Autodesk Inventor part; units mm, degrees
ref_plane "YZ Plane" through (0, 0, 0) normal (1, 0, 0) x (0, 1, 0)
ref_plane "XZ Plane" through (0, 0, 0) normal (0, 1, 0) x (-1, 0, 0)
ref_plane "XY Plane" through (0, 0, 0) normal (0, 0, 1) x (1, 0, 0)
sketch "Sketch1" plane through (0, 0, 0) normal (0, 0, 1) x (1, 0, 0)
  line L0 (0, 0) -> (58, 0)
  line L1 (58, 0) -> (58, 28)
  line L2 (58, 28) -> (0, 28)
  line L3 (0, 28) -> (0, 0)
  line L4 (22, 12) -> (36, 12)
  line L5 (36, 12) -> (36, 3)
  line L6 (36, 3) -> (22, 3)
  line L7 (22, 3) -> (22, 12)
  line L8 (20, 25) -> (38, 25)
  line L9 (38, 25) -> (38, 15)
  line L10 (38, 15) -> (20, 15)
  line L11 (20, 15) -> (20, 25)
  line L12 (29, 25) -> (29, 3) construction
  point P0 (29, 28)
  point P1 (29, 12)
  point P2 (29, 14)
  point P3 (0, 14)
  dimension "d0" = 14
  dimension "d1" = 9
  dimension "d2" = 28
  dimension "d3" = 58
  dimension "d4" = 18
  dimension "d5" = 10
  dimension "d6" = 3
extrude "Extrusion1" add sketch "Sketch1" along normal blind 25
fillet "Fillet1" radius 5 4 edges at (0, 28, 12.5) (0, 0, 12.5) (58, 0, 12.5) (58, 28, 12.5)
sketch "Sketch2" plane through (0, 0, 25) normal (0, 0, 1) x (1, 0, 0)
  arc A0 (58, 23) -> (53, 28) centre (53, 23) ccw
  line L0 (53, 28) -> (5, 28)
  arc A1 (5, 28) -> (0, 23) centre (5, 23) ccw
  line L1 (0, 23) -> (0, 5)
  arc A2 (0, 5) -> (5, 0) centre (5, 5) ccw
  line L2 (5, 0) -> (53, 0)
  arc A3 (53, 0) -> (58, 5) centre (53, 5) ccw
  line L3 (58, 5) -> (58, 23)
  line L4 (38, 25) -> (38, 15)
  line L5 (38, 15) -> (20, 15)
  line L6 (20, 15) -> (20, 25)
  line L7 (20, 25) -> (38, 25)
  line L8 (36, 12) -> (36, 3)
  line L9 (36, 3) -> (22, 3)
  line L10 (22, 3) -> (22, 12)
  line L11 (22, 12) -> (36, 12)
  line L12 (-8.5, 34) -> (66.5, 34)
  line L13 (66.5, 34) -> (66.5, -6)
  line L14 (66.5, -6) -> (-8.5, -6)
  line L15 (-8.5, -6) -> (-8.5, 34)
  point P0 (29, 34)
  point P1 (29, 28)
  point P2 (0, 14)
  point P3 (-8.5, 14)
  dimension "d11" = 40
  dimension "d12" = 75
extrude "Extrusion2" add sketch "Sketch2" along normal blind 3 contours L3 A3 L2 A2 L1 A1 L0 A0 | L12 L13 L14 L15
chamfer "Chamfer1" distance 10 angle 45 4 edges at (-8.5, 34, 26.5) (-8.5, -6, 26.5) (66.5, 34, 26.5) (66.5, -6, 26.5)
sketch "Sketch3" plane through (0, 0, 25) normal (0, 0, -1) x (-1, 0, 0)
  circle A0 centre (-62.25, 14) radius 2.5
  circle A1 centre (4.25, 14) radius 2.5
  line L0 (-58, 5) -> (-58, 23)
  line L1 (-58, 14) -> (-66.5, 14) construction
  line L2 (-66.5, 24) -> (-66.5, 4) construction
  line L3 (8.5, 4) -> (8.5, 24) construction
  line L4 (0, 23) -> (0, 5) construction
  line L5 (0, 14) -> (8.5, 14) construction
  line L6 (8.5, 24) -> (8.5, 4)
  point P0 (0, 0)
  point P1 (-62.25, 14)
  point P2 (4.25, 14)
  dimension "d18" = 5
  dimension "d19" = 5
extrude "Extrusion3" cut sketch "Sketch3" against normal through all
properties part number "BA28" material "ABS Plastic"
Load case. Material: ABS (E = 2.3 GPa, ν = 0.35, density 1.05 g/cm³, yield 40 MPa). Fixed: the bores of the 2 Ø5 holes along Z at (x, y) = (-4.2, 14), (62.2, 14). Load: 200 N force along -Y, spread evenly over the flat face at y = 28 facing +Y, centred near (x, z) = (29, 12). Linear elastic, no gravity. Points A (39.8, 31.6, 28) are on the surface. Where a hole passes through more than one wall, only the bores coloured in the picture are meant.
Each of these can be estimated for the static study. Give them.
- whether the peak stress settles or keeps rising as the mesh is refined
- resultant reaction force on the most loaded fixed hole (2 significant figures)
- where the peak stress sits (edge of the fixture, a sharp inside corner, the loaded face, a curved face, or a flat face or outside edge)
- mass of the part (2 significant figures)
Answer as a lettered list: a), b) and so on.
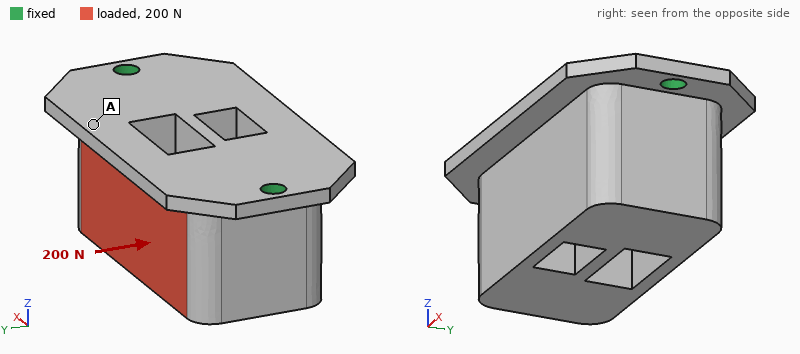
a) keeps rising
b) 100 N
c) edge of the fixture
d) 42 g
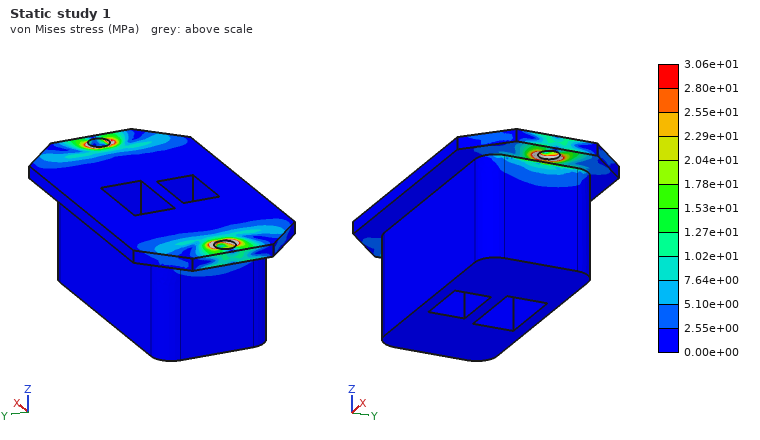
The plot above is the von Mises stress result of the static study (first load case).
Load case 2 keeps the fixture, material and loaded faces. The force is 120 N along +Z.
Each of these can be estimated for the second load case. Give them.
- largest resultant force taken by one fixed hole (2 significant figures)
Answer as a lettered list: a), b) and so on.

a) 72 N
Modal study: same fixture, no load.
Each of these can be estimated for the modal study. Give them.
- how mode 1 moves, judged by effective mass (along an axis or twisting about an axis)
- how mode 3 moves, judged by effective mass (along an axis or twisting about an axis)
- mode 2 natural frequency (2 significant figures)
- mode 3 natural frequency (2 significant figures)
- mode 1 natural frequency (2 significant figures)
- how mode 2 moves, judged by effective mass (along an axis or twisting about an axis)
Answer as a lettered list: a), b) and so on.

a) along Y
b) along X
c) 2000 Hz
d) 2600 Hz
e) 480 Hz
f) along Z
